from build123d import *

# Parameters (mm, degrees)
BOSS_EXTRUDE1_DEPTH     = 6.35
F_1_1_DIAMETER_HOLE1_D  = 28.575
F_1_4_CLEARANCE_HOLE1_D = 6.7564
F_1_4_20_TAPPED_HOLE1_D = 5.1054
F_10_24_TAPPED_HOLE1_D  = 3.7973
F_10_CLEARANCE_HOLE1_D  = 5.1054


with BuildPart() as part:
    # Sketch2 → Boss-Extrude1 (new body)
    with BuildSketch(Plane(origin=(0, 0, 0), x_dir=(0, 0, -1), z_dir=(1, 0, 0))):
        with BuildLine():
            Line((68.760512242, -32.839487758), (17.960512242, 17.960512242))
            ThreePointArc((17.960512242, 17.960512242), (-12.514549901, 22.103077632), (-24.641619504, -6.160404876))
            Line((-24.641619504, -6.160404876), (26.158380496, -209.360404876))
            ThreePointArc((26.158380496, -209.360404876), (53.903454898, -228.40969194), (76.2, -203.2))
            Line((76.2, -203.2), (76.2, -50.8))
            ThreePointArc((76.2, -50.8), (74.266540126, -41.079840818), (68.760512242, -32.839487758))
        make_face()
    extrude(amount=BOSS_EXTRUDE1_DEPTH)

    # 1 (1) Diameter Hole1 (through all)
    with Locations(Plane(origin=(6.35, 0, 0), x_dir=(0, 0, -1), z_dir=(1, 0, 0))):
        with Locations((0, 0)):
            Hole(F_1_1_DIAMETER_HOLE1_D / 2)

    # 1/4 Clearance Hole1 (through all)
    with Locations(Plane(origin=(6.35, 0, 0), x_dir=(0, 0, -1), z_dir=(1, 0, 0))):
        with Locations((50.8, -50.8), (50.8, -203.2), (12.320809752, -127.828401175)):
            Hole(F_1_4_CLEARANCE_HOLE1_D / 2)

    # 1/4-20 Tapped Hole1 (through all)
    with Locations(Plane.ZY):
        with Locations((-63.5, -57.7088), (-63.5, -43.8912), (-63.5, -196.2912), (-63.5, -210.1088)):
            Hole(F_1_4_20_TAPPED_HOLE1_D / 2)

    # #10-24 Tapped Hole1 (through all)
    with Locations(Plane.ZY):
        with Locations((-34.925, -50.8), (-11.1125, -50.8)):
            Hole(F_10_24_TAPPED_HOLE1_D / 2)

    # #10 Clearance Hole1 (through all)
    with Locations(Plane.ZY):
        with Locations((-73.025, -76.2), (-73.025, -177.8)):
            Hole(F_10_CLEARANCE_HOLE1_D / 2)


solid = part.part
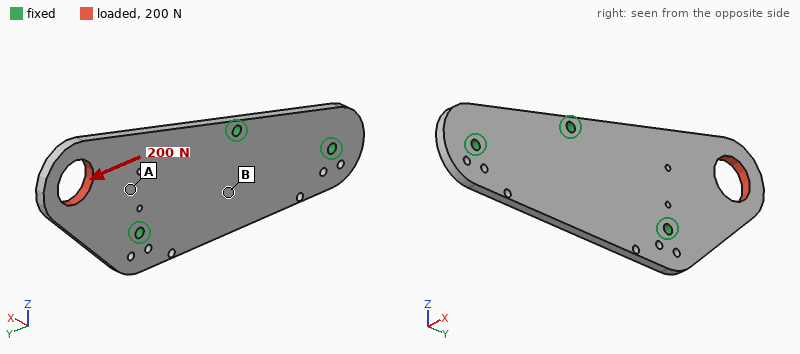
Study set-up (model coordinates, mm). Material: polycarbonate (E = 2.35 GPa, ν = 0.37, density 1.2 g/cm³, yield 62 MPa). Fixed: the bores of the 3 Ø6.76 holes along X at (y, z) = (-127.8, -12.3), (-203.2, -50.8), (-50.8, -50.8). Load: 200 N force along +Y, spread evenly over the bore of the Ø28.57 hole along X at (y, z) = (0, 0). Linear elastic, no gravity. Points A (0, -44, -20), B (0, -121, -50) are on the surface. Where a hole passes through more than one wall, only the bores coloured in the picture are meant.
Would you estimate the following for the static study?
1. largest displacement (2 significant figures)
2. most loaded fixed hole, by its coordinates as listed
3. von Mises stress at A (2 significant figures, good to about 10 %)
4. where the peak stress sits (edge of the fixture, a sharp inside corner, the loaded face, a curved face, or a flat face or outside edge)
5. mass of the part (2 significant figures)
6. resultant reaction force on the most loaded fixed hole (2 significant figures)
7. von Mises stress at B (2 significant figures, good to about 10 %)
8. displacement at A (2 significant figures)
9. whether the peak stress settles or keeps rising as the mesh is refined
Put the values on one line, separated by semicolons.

0.11 mm; (-127.8, -12.3); 0.55 MPa; edge of the fixture; 120 g; 130 N; 0.26 MPa; 0.022 mm; keeps rising
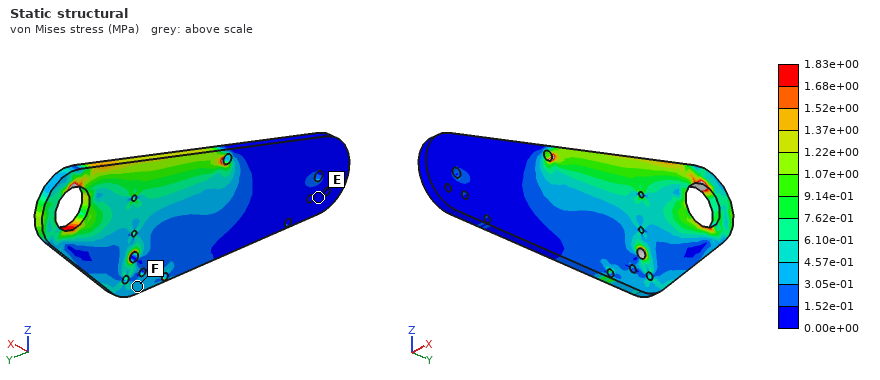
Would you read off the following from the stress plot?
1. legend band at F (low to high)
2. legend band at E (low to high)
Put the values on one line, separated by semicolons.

3.05e-01 to 4.57e-01 MPa; 0.00e+00 to 1.52e-01 MPa
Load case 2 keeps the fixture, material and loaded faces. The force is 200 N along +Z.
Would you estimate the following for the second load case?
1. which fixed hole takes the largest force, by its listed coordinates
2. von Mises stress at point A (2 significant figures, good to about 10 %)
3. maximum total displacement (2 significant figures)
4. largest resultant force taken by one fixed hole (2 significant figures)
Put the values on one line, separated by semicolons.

(-50.8, -50.8); 0.86 MPa; 0.17 mm; 290 N
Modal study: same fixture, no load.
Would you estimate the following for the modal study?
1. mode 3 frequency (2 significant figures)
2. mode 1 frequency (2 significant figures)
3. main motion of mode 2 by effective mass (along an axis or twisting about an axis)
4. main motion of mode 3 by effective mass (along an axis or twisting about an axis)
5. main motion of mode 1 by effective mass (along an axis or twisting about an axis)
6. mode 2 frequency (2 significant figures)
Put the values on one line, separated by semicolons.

550 Hz; 210 Hz; twisting about Y; along X; along X; 480 Hz
